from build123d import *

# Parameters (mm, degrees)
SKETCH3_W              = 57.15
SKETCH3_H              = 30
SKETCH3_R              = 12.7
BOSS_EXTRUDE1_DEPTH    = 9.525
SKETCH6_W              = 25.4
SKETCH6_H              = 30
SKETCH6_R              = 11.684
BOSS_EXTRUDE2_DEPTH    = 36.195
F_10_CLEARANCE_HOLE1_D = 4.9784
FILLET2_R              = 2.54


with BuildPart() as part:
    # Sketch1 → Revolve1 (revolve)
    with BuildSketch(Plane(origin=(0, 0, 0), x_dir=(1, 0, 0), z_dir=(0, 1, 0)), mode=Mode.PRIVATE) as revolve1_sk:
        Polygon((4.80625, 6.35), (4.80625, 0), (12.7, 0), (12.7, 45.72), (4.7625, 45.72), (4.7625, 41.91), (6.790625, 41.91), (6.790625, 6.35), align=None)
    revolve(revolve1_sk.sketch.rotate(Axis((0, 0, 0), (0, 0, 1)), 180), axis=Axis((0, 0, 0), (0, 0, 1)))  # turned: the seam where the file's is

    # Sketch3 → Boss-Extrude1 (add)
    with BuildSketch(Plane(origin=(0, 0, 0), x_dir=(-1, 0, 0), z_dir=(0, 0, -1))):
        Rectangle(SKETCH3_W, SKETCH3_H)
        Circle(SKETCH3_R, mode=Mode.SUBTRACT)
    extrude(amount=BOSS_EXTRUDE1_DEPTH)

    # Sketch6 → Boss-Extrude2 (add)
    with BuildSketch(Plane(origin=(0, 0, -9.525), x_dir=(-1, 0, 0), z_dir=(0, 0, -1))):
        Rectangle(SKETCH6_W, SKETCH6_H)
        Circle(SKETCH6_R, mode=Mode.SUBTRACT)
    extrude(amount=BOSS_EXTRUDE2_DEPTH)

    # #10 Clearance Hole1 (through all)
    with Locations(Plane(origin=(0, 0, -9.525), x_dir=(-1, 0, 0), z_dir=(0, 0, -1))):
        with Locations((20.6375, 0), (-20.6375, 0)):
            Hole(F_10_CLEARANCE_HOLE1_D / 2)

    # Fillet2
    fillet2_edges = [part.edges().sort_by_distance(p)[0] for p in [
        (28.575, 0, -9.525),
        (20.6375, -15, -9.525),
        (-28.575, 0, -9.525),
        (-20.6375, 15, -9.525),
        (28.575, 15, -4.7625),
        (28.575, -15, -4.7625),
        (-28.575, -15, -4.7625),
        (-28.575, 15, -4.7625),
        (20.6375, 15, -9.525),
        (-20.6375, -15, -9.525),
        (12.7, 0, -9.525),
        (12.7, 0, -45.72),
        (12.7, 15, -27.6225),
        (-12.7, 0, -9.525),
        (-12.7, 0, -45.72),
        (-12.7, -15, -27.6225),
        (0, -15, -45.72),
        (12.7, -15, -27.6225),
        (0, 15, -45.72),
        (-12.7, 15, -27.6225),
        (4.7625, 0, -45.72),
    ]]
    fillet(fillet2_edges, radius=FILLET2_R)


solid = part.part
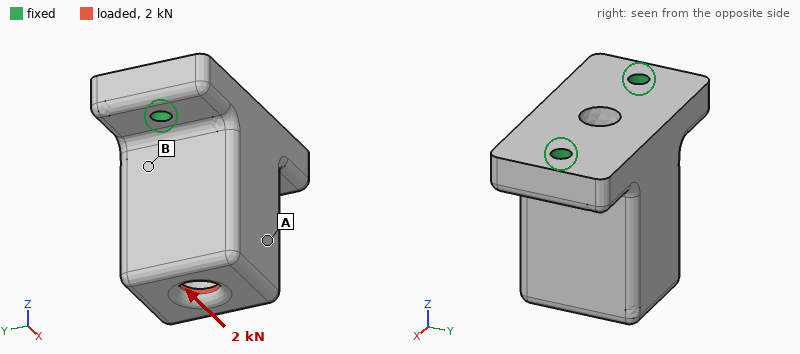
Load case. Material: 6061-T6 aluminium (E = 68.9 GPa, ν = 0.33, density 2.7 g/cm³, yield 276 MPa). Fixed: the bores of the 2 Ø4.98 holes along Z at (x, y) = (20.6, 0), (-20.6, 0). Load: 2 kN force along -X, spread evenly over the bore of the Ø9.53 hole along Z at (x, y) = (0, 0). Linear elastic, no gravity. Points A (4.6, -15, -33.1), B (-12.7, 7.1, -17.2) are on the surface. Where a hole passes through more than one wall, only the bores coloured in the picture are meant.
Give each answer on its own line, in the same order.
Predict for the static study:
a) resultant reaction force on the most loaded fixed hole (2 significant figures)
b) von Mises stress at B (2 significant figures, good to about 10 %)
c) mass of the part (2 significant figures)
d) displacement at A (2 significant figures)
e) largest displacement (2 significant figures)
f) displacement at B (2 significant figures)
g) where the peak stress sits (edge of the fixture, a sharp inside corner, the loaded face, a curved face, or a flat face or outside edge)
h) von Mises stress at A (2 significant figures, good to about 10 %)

2.3 kN
18 MPa
100 g
21 µm
37 µm
11 µm
the loaded face
8.5 MPa
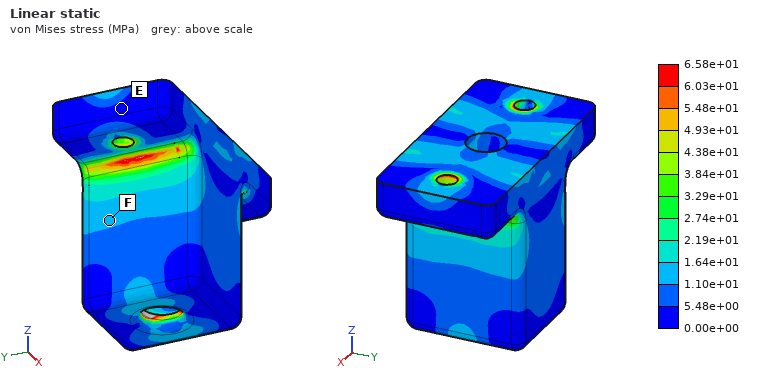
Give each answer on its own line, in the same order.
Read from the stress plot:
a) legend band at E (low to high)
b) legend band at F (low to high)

0.00e+00 to 5.48e+00 MPa
1.10e+01 to 1.64e+01 MPa
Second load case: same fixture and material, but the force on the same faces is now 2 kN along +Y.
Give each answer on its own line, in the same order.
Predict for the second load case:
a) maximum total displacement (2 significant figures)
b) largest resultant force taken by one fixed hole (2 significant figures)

0.12 mm
1.0 kN
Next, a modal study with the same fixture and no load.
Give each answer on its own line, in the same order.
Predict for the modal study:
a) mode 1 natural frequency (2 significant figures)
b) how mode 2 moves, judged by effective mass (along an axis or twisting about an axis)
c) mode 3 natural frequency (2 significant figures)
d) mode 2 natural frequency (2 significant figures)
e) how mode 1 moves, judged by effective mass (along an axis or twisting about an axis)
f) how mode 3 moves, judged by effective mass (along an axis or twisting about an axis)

3900 Hz
along X
12 kHz
7900 Hz
along Y
along Z
